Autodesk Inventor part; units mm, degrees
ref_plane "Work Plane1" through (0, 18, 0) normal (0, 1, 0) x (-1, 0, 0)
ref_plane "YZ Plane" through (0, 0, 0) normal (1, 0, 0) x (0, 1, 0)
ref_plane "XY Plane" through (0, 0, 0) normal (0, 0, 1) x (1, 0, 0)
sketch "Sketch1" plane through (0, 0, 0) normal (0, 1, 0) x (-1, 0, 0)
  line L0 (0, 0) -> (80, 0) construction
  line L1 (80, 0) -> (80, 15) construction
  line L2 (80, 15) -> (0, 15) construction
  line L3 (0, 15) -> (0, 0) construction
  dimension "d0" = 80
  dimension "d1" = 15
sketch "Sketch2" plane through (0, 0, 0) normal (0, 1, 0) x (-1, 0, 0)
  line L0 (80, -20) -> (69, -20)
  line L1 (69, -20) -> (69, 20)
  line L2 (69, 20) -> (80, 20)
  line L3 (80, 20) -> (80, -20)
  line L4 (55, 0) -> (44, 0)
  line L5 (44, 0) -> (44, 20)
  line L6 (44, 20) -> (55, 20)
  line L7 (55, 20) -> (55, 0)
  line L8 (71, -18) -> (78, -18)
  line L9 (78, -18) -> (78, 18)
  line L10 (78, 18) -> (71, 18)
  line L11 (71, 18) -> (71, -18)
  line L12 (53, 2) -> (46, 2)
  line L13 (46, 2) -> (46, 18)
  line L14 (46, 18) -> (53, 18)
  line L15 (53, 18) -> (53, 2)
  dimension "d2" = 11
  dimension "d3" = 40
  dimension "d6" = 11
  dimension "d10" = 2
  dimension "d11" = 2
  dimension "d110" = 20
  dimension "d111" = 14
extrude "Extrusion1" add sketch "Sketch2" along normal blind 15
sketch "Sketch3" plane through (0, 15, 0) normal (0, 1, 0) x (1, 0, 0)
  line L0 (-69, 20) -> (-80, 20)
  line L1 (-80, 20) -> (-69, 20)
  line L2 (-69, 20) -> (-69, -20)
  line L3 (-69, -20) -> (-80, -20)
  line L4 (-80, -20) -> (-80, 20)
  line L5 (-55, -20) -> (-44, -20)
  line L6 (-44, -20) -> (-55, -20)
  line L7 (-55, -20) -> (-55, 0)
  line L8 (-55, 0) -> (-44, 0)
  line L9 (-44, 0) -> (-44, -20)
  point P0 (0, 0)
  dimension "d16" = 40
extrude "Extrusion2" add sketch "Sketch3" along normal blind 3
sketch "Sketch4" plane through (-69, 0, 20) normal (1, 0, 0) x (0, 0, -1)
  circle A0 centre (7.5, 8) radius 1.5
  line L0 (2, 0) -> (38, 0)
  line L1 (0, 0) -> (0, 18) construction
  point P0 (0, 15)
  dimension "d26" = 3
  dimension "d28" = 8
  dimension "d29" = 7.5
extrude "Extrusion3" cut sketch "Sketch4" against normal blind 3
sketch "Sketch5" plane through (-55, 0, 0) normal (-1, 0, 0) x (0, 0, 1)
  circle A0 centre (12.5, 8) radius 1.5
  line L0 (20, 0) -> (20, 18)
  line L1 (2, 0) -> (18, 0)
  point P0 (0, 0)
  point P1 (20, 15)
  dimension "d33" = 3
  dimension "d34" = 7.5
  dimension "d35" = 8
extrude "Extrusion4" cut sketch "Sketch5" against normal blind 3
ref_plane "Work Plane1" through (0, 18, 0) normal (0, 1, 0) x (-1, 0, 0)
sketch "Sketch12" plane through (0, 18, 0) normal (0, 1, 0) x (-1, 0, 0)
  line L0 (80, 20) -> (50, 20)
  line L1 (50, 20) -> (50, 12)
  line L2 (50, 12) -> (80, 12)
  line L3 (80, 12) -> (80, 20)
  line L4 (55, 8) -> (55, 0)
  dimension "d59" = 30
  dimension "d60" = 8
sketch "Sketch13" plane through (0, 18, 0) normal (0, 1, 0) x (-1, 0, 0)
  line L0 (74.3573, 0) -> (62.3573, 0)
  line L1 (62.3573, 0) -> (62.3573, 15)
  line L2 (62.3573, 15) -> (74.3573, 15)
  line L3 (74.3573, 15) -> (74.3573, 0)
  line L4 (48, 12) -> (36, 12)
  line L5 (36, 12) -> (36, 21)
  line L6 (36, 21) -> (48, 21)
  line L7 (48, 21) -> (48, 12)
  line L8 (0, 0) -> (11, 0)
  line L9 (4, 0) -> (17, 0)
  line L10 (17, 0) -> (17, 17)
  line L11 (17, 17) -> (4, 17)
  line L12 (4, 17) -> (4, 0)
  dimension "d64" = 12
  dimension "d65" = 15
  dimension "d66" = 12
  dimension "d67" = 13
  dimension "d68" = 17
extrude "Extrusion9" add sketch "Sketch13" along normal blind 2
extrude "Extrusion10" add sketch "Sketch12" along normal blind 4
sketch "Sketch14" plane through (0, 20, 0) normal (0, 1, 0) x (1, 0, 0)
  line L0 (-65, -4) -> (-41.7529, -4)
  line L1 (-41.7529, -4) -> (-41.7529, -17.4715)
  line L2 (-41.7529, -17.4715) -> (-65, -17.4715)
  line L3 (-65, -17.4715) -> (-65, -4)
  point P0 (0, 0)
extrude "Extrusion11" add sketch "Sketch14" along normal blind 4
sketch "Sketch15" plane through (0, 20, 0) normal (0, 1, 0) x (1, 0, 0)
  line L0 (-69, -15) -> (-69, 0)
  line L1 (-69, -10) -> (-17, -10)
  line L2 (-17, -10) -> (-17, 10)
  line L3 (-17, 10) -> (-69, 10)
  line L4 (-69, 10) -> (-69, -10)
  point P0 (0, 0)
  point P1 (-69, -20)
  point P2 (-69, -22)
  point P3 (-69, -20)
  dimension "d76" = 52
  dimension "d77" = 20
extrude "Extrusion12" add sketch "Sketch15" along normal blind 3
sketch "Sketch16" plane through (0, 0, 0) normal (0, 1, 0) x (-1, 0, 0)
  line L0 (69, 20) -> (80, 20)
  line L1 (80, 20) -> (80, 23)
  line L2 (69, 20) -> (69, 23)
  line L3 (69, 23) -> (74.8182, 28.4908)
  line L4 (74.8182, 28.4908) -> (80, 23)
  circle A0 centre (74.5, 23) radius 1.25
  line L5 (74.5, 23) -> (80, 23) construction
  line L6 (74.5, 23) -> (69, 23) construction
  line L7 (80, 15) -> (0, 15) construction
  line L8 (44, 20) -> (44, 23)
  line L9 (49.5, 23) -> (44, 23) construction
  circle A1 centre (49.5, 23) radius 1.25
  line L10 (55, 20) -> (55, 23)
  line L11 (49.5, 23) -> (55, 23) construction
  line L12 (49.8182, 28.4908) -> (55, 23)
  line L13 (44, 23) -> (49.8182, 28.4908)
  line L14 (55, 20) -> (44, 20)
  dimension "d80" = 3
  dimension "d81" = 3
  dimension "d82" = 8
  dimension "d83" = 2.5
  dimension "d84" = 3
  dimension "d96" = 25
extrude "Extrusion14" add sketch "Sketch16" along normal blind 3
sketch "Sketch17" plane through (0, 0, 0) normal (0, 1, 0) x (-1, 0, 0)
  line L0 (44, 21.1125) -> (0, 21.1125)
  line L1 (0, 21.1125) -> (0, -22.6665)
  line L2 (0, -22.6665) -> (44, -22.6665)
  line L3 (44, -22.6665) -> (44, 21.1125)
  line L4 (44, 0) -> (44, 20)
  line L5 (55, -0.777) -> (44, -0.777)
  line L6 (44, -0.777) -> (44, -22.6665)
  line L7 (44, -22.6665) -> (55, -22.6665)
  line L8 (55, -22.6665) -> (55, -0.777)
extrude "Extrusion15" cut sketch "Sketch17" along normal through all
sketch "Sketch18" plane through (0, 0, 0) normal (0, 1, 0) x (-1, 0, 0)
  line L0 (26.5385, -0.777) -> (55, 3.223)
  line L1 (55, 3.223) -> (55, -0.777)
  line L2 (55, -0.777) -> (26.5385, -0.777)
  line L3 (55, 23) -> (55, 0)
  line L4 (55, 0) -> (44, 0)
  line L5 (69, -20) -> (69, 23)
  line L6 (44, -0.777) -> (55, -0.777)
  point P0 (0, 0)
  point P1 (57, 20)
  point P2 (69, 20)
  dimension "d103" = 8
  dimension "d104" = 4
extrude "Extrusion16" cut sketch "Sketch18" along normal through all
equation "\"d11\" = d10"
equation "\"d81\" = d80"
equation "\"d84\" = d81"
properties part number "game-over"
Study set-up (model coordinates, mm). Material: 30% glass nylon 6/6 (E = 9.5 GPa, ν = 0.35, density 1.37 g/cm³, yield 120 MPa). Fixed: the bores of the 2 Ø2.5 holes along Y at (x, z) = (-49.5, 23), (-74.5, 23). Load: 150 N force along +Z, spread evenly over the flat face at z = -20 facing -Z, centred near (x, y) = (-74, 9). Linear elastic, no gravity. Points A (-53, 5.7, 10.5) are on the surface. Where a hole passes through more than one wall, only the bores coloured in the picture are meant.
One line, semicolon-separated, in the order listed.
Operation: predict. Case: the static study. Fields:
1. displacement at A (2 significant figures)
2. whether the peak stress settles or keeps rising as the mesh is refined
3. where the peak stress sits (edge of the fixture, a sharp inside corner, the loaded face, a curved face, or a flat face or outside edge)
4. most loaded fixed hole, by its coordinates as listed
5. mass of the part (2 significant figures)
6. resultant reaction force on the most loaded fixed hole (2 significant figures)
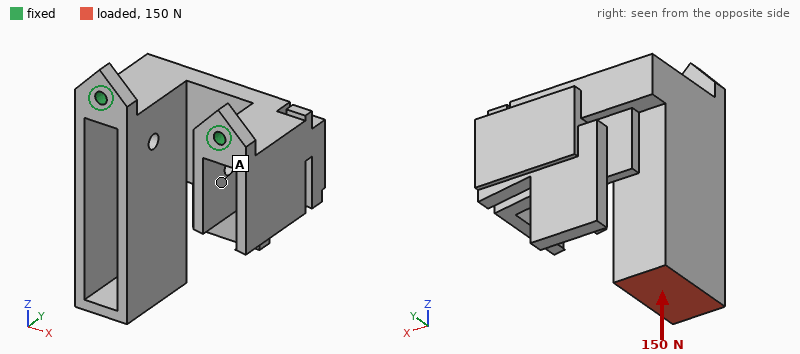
0.14 mm; keeps rising; edge of the fixture; (-74.5, 23); 13 g; 140 N
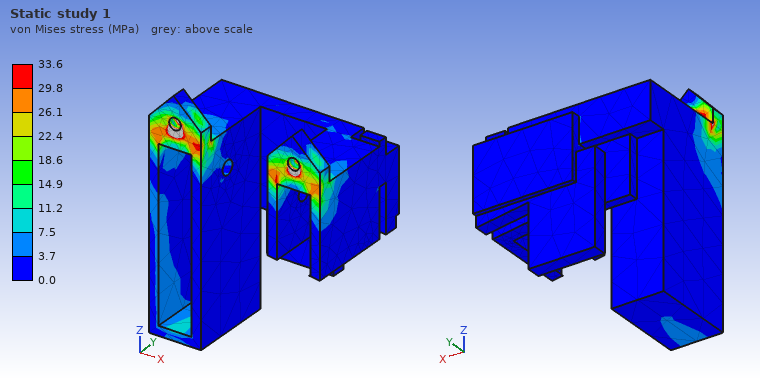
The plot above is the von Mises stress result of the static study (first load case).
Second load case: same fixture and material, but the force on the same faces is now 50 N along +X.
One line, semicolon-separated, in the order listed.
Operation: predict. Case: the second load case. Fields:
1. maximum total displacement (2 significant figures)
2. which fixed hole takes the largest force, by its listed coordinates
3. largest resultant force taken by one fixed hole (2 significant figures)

0.72 mm; (-74.5, 23); 56 N
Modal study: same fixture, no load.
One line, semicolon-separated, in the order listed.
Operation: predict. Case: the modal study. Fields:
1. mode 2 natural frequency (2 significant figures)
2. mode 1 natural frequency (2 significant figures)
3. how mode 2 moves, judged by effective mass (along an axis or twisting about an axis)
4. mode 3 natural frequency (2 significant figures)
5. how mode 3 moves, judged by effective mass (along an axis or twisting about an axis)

980 Hz; 520 Hz; along X; 2500 Hz; along X
